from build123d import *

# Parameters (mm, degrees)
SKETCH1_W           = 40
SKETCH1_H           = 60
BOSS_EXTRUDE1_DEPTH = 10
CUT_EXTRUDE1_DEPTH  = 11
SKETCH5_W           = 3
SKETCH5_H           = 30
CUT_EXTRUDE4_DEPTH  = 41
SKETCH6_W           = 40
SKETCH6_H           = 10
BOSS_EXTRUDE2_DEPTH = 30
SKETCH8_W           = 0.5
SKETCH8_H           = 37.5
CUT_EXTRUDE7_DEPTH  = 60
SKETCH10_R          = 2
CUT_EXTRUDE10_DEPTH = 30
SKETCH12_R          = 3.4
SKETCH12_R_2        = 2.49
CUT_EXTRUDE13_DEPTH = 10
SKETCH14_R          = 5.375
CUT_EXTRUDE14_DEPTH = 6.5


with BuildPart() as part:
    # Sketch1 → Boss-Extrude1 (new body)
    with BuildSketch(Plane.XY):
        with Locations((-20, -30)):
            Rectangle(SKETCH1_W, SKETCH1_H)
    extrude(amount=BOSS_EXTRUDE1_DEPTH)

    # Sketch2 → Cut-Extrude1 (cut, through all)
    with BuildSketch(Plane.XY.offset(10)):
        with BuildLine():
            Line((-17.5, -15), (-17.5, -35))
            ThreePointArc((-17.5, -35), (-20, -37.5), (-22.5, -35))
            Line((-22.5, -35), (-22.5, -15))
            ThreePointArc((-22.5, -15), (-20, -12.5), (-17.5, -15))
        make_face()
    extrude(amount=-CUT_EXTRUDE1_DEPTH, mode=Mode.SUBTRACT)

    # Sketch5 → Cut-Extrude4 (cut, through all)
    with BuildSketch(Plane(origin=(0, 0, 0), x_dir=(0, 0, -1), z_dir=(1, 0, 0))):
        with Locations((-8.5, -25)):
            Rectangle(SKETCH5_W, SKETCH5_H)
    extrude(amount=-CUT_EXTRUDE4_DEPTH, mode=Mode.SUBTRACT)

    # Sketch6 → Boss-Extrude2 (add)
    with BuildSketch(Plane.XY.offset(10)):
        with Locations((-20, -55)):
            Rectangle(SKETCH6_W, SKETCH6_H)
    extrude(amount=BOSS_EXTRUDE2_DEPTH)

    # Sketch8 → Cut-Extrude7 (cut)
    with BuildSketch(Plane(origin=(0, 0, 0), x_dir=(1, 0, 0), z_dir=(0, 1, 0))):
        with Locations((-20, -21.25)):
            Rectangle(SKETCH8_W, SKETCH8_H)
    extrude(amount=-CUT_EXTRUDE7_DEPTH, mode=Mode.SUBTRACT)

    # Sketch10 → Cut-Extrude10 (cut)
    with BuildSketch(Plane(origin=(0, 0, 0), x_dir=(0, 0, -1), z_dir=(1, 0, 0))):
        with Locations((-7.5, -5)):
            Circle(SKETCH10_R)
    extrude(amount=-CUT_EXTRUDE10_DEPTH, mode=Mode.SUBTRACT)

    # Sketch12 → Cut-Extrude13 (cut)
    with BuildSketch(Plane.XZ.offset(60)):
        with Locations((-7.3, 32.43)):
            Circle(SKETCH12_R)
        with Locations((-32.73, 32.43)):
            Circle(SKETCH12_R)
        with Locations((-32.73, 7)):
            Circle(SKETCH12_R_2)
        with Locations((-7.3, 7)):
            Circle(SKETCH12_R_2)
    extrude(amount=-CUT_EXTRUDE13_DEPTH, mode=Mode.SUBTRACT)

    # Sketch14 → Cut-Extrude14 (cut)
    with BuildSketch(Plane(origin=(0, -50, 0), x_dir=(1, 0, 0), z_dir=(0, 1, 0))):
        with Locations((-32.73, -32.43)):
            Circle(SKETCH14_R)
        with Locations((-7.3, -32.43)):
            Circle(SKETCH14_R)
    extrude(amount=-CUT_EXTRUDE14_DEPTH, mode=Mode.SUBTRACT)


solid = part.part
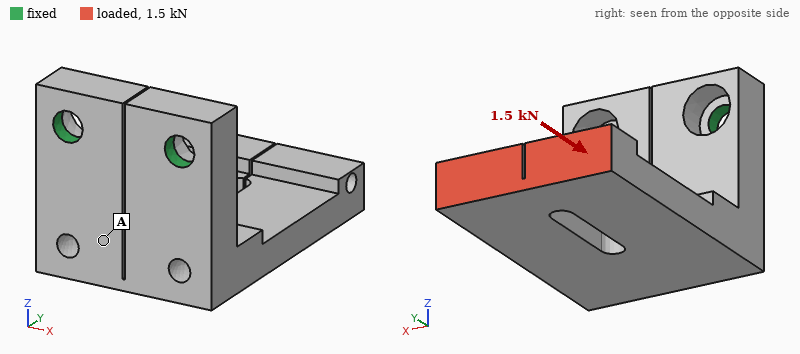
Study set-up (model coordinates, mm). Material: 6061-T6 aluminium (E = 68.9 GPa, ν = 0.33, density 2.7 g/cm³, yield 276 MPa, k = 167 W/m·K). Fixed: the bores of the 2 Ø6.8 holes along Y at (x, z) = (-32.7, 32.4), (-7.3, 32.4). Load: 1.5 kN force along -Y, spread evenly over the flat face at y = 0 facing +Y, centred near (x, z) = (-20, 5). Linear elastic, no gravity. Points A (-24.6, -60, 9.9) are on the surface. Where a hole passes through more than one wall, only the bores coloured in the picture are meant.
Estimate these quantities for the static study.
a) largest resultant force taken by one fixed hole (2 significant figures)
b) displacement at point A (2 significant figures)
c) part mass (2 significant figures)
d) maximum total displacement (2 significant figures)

750 N
0.11 mm
79 g
0.36 mm
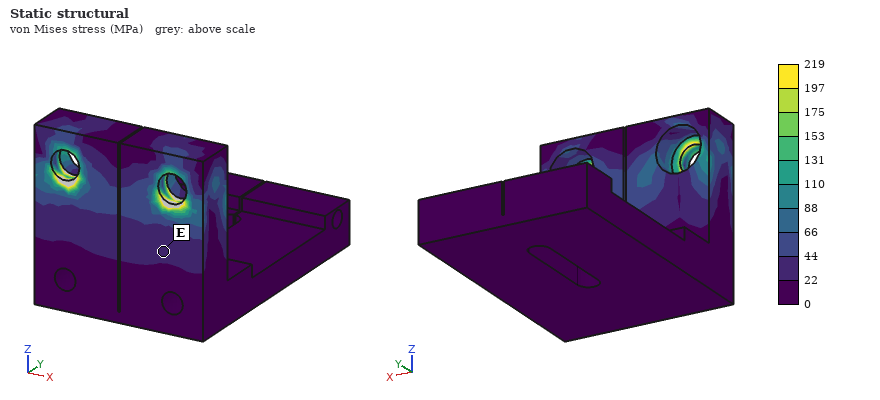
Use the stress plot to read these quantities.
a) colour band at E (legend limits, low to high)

22 to 44 MPa
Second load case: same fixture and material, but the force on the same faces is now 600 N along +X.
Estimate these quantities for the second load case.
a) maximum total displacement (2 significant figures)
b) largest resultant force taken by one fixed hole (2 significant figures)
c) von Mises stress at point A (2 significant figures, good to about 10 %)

0.24 mm
990 N
28 MPa
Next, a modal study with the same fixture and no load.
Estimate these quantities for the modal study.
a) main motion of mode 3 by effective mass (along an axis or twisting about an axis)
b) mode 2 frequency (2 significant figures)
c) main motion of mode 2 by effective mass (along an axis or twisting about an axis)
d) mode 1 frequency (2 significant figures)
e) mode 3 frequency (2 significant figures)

along Y
2000 Hz
along X
1200 Hz
3600 Hz
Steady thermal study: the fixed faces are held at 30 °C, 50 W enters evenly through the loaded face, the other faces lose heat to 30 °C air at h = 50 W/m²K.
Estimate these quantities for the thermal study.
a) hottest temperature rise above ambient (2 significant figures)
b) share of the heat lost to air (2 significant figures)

66 K
30 %
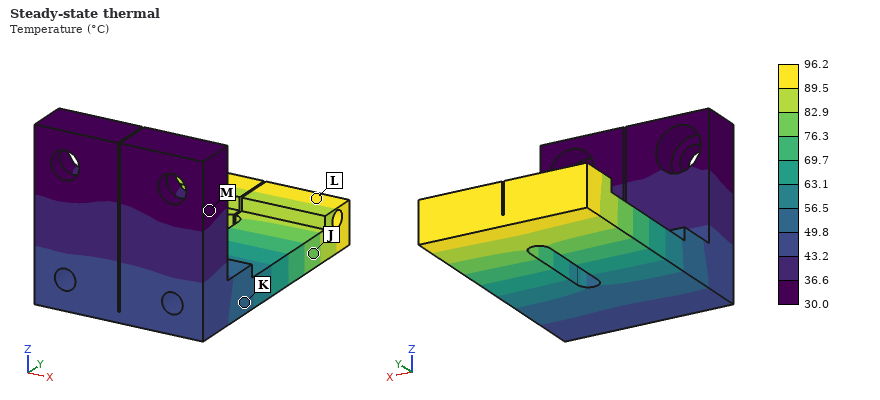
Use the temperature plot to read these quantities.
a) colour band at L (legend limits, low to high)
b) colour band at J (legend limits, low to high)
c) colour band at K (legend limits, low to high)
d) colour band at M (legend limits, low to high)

89.5 to 96.2 °C
76.3 to 82.9 °C
49.8 to 56.5 °C
30.0 to 36.6 °C
